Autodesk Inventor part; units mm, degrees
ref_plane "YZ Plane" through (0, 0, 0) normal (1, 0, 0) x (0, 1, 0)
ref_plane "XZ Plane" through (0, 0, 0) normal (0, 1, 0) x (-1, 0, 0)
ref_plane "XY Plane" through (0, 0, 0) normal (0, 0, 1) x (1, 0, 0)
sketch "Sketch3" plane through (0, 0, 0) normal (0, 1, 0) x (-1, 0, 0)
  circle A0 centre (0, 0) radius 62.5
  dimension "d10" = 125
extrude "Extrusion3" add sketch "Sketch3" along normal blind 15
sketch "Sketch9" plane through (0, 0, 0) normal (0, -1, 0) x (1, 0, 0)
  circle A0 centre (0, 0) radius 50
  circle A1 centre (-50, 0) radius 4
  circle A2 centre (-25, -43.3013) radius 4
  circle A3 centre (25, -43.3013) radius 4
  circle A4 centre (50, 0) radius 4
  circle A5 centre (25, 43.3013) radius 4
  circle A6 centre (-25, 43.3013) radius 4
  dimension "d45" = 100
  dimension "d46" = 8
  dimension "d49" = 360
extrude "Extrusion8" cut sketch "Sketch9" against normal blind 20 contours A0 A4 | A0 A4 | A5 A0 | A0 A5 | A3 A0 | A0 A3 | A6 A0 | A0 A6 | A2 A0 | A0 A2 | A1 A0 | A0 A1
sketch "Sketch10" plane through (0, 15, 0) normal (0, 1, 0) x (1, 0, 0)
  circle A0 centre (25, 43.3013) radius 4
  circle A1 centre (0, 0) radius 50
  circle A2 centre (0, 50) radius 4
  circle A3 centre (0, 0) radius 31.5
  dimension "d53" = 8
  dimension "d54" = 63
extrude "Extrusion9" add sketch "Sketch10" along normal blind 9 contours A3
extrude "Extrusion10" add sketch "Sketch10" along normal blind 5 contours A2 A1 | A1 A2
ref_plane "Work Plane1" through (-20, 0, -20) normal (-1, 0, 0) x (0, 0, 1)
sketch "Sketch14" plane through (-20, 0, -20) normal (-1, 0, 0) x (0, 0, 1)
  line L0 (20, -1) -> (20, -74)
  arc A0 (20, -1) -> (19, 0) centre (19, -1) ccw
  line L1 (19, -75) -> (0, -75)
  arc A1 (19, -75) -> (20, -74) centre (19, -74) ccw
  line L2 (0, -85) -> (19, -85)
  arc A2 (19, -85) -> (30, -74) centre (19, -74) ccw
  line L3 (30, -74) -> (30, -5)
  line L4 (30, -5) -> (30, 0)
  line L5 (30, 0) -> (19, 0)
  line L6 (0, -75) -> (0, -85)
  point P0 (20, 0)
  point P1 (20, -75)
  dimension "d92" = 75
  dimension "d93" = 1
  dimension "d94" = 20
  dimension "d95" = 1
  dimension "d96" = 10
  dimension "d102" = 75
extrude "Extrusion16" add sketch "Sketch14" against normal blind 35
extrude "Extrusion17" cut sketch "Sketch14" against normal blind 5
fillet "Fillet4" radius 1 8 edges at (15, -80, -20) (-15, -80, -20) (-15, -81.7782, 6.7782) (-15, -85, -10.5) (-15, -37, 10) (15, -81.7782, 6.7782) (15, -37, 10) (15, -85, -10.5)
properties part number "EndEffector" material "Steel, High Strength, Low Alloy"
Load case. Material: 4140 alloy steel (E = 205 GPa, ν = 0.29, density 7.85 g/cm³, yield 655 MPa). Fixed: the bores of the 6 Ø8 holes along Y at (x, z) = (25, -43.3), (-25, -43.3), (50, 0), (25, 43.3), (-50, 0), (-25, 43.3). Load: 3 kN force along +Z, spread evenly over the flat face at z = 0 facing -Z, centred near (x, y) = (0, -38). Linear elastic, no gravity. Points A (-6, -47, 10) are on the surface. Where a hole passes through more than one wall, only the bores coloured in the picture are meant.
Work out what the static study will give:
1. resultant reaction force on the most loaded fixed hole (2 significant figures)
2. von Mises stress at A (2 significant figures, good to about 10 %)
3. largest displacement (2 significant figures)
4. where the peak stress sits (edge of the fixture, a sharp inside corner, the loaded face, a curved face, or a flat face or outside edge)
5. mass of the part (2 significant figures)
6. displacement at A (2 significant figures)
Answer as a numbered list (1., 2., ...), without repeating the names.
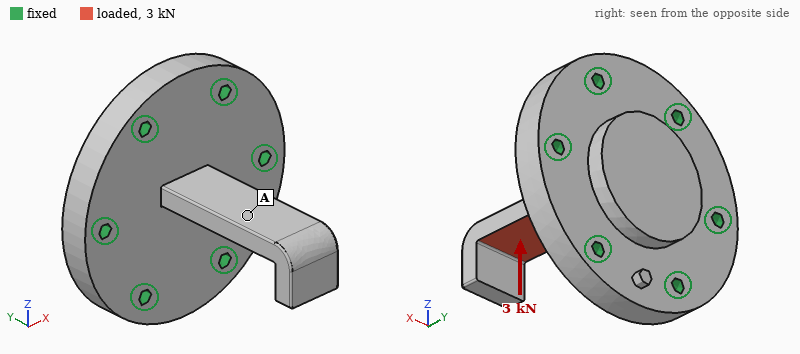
1. 1.3 kN
2. 30 MPa
3. 0.45 mm
4. the loaded face
5. 1.9 kg
6. 0.20 mm
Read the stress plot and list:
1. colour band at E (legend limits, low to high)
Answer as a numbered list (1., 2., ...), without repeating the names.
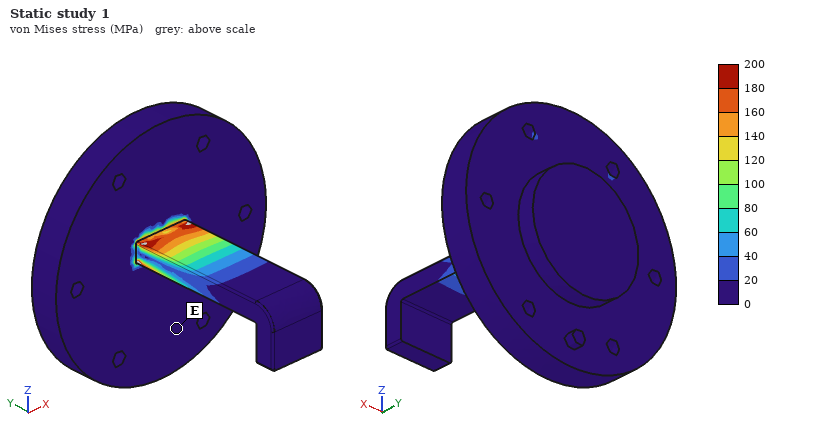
1. 0 to 20 MPa
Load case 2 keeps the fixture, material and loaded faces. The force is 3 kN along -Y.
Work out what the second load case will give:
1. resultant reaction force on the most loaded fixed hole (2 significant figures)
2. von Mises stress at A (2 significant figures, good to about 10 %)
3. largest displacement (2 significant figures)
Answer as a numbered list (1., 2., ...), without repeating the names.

1. 560 N
2. 7.4 MPa
3. 80 µm
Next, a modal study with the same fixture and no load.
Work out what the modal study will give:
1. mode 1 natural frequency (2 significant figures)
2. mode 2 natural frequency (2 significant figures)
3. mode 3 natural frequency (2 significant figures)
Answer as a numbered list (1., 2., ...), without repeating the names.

1. 810 Hz
2. 2000 Hz
3. 3800 Hz
